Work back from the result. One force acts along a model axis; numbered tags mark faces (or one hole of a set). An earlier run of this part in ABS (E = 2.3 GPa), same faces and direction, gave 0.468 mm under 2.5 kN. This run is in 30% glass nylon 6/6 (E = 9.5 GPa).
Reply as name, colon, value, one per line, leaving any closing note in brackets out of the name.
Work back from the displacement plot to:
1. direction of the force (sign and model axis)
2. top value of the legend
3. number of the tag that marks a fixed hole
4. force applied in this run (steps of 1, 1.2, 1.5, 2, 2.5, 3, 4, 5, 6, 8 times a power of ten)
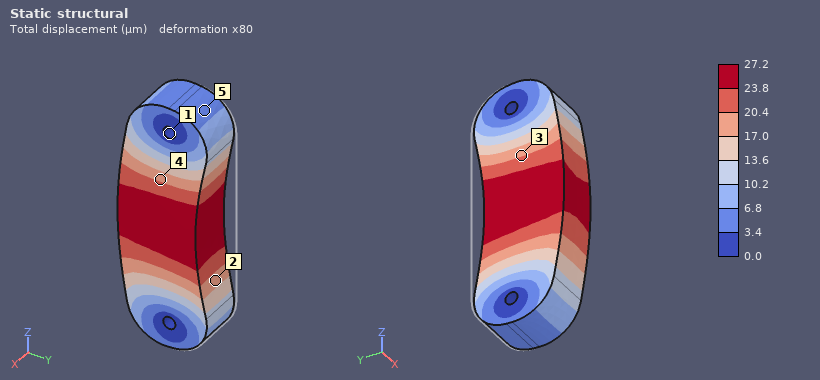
direction of the force: -Y
top value of the legend: 27.2 µm
number of the tag that marks a fixed hole: 1
force applied in this run: 600 N
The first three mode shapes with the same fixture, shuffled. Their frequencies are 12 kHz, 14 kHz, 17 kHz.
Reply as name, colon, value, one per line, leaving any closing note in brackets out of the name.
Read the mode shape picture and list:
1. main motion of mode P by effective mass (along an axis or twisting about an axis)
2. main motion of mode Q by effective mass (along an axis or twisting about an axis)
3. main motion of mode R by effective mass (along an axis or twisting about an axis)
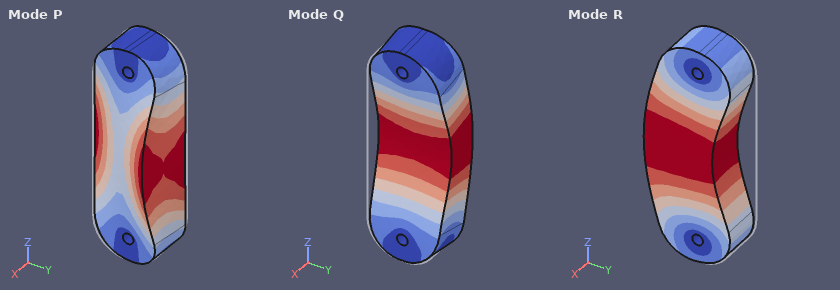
main motion of mode P by effective mass: twisting about Z
main motion of mode Q by effective mass: along X
main motion of mode R by effective mass: along Y
